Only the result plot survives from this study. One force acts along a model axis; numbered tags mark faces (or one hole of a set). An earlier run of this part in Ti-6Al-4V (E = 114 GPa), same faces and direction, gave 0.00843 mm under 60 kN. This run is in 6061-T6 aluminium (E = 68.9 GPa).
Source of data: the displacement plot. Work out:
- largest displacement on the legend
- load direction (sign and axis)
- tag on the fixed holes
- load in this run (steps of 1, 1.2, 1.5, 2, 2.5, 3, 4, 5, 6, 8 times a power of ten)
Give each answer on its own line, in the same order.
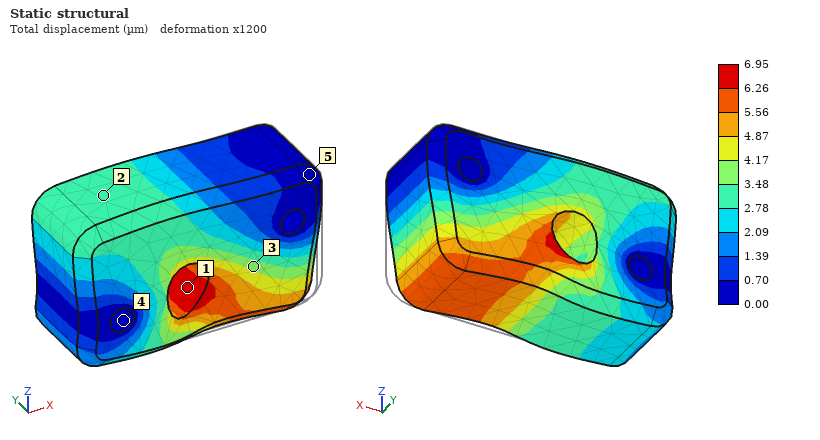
6.95 µm
-X
4
30 kN
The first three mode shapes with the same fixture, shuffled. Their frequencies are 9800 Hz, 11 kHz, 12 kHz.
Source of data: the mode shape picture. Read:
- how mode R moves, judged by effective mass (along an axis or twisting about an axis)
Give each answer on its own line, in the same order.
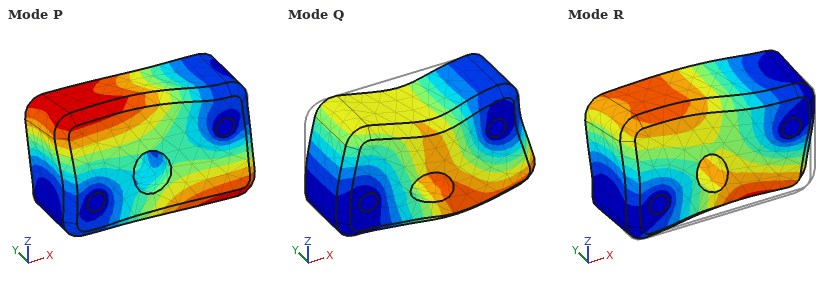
along Y
